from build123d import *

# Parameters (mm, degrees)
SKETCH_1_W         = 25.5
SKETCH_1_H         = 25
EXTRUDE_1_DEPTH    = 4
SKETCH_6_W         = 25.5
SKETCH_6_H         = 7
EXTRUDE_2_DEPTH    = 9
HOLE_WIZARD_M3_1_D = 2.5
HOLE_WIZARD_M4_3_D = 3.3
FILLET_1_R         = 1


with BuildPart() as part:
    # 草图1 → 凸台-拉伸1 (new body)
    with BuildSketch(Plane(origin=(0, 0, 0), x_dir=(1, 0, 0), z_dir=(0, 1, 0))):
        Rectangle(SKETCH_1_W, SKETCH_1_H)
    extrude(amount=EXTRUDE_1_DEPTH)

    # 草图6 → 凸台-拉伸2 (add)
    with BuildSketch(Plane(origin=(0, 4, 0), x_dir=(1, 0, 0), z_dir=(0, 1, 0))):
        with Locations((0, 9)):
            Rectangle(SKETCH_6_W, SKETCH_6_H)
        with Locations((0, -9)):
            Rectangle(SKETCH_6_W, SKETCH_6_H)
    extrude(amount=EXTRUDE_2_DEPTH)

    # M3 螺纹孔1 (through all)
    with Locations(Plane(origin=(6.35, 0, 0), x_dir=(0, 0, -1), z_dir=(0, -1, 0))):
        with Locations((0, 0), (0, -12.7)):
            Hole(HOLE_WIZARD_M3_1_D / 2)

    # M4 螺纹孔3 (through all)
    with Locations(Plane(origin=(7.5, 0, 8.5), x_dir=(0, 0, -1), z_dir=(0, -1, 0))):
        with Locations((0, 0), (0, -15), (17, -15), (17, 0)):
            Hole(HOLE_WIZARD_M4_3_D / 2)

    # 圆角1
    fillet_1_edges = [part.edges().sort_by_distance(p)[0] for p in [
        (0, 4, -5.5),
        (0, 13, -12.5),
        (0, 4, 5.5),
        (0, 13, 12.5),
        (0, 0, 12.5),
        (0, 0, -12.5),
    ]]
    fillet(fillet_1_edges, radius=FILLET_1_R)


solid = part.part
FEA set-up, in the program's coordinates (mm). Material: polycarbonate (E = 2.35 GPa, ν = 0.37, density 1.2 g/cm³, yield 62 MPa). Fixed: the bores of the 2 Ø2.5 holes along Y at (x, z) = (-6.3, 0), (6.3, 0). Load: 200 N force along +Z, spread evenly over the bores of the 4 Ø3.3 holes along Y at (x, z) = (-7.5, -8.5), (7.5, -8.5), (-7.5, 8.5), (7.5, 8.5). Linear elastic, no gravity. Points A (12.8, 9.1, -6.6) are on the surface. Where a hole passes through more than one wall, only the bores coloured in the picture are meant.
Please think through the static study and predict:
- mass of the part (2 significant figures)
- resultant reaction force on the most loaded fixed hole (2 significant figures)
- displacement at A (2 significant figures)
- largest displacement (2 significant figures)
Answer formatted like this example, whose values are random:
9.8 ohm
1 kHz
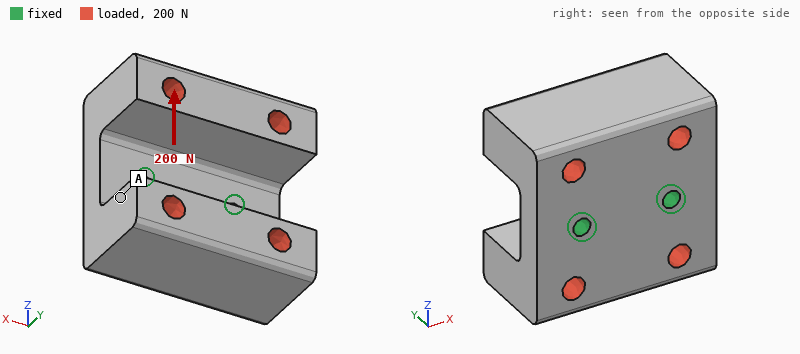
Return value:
6.3 g
100 N
0.099 mm
0.17 mm
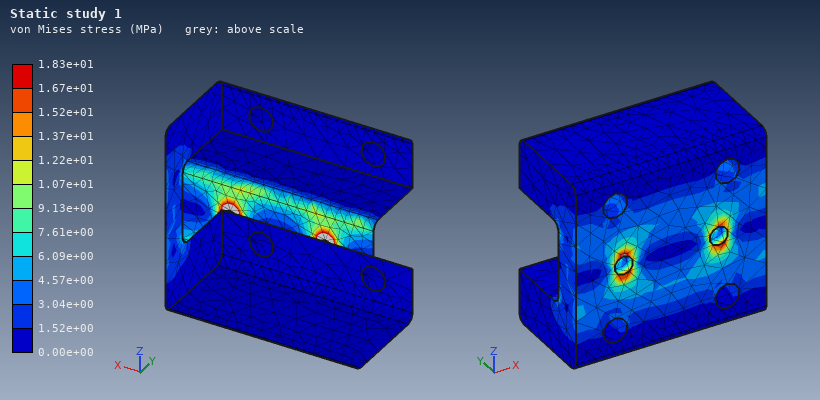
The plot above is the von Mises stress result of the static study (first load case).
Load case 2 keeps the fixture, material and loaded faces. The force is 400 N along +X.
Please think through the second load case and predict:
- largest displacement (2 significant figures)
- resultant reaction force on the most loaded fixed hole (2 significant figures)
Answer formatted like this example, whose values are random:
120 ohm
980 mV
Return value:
89 µm
230 N
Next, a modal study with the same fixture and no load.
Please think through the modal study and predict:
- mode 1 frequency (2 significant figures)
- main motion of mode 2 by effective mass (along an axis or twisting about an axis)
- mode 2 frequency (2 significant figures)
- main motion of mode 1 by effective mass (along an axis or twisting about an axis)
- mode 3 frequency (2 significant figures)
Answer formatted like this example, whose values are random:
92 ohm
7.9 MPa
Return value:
2200 Hz
along Y
2700 Hz
along Z
4400 Hz
